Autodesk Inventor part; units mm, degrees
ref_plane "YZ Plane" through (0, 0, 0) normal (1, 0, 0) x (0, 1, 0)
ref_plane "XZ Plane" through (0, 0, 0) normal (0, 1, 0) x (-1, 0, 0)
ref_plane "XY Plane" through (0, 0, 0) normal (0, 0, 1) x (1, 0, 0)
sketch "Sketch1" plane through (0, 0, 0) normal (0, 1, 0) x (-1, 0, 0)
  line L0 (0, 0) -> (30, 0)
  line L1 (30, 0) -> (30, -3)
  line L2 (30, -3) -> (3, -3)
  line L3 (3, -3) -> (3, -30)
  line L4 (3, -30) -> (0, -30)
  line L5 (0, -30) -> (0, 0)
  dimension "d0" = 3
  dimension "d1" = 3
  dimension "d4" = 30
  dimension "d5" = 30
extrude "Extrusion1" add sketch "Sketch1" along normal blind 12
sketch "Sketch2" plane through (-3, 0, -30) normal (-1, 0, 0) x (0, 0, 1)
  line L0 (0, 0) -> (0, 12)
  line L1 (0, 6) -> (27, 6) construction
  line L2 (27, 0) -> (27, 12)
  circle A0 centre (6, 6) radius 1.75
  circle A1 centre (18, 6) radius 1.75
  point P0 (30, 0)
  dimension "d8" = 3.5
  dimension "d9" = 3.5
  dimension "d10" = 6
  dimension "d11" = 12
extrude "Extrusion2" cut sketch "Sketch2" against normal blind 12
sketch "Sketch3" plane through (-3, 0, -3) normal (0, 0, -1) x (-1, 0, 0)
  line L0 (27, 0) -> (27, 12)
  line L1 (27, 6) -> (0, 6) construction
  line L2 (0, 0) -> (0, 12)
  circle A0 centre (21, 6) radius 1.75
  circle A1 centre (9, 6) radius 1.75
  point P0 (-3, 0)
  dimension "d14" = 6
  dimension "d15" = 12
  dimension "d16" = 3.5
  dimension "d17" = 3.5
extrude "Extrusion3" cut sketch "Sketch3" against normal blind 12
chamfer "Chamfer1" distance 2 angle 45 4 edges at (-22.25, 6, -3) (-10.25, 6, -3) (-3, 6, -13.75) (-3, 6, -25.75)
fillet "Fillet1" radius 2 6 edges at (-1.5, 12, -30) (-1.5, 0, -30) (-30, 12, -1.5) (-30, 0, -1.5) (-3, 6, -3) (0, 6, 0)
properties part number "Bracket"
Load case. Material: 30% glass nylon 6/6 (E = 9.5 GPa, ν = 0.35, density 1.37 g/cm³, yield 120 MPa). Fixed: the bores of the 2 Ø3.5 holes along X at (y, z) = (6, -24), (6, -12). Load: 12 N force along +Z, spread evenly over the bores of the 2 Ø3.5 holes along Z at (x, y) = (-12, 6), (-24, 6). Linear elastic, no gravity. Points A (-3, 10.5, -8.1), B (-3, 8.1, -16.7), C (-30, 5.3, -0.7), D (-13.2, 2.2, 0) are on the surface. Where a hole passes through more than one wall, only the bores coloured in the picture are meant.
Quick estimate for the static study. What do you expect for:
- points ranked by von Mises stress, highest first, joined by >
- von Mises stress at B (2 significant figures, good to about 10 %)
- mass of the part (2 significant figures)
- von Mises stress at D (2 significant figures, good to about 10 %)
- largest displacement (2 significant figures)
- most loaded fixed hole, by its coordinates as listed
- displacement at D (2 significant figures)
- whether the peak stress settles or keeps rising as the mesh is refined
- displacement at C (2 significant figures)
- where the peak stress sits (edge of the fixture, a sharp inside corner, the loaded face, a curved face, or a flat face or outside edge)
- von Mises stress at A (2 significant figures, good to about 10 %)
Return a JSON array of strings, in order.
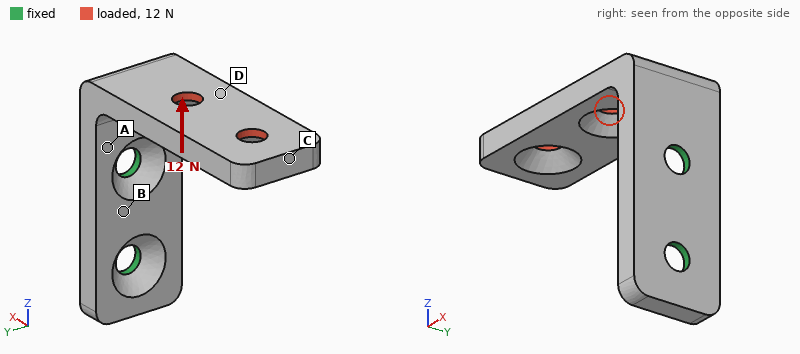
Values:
["A > D > B > C", "3.0 MPa", "2.5 g", "5.2 MPa", "0.43 mm", "(6, -24)", "0.17 mm", "keeps rising", "0.43 mm", "edge of the fixture", "14 MPa"]
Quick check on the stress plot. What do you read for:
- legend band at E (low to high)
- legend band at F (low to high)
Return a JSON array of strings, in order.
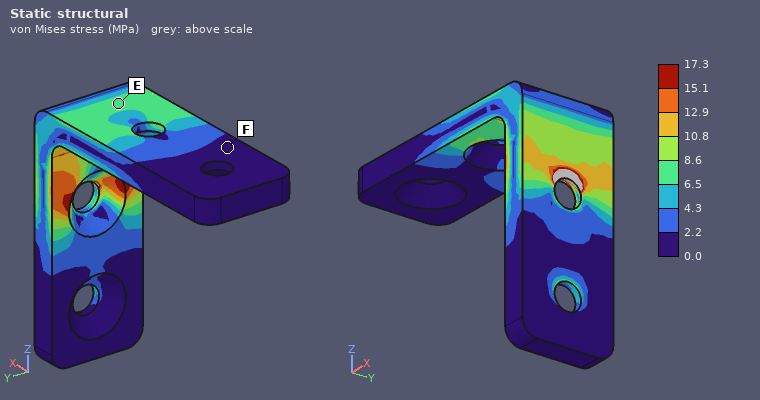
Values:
["6.5 to 8.6 MPa", "0.0 to 2.2 MPa"]
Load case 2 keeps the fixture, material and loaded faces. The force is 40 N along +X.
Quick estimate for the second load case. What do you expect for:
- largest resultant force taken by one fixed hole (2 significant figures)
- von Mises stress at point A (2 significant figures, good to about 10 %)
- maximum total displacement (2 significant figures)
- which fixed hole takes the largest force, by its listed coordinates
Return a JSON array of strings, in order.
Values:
["83 N", "22 MPa", "0.49 mm", "(6, -12)"]
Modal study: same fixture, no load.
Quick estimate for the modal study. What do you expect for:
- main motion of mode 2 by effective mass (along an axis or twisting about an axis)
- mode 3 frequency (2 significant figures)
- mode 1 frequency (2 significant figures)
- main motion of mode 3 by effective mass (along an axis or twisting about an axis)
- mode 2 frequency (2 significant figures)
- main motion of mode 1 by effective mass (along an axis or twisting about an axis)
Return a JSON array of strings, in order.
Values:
["along Y", "3700 Hz", "990 Hz", "along X", "1300 Hz", "along Z"]
